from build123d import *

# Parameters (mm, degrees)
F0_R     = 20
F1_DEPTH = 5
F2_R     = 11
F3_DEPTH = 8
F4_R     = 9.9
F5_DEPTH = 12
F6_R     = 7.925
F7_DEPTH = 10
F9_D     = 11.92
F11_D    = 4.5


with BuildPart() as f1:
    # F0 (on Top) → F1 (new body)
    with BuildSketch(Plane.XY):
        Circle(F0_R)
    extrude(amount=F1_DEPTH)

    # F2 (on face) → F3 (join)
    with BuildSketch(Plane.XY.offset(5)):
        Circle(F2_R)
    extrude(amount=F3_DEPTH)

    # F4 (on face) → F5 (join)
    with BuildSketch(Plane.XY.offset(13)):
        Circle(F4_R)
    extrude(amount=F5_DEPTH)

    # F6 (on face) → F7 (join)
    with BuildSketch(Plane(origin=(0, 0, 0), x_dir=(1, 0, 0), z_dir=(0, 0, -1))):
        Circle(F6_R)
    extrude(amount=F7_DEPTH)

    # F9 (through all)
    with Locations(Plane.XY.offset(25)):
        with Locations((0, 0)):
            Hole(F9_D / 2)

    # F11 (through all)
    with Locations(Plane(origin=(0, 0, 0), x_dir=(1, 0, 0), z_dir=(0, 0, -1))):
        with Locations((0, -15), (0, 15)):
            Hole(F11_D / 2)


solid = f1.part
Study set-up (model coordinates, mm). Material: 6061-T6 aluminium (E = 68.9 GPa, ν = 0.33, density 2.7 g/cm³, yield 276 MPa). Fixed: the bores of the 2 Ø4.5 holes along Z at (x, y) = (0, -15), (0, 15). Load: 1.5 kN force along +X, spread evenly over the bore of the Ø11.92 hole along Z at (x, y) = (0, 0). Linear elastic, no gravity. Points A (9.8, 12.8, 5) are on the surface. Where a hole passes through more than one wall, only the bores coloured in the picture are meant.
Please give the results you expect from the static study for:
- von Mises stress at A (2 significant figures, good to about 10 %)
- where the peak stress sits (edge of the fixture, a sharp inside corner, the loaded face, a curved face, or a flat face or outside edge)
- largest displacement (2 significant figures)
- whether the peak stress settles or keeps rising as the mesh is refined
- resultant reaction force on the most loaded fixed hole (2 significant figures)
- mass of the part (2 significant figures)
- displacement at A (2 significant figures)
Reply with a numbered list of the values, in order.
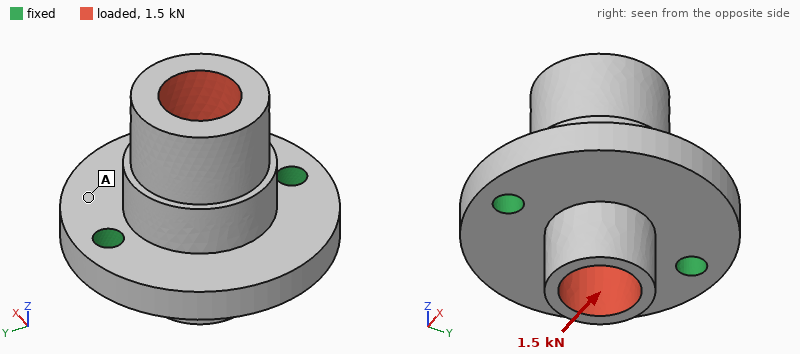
1. 11 MPa
2. edge of the fixture
3. 30 µm
4. keeps rising
5. 750 N
6. 30 g
7. 7.8 µm
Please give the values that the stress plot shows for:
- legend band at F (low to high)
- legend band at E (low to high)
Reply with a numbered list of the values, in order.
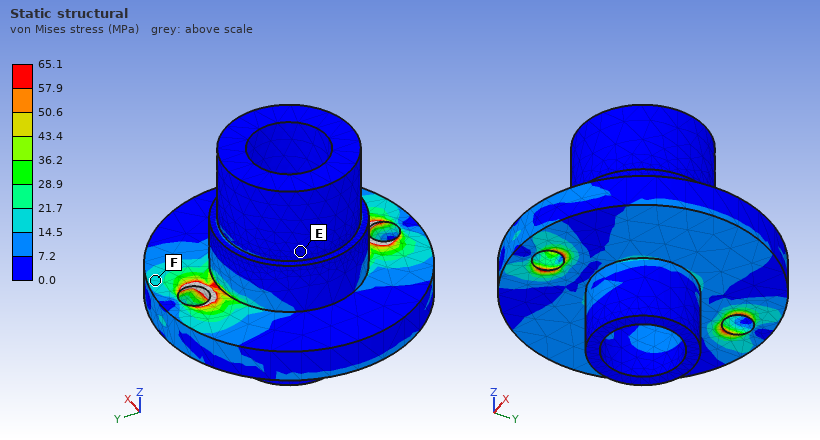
1. 14.5 to 21.7 MPa
2. 0.0 to 7.2 MPa
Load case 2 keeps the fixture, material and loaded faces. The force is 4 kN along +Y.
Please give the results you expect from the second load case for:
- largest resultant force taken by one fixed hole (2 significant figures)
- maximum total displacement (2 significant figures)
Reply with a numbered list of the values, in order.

1. 2.1 kN
2. 19 µm
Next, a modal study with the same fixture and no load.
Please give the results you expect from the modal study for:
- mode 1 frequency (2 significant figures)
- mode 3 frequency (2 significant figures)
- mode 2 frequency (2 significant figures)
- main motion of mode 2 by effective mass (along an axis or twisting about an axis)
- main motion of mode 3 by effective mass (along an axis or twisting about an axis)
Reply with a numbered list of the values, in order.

1. 6500 Hz
2. 18 kHz
3. 16 kHz
4. along Z
5. along Y
